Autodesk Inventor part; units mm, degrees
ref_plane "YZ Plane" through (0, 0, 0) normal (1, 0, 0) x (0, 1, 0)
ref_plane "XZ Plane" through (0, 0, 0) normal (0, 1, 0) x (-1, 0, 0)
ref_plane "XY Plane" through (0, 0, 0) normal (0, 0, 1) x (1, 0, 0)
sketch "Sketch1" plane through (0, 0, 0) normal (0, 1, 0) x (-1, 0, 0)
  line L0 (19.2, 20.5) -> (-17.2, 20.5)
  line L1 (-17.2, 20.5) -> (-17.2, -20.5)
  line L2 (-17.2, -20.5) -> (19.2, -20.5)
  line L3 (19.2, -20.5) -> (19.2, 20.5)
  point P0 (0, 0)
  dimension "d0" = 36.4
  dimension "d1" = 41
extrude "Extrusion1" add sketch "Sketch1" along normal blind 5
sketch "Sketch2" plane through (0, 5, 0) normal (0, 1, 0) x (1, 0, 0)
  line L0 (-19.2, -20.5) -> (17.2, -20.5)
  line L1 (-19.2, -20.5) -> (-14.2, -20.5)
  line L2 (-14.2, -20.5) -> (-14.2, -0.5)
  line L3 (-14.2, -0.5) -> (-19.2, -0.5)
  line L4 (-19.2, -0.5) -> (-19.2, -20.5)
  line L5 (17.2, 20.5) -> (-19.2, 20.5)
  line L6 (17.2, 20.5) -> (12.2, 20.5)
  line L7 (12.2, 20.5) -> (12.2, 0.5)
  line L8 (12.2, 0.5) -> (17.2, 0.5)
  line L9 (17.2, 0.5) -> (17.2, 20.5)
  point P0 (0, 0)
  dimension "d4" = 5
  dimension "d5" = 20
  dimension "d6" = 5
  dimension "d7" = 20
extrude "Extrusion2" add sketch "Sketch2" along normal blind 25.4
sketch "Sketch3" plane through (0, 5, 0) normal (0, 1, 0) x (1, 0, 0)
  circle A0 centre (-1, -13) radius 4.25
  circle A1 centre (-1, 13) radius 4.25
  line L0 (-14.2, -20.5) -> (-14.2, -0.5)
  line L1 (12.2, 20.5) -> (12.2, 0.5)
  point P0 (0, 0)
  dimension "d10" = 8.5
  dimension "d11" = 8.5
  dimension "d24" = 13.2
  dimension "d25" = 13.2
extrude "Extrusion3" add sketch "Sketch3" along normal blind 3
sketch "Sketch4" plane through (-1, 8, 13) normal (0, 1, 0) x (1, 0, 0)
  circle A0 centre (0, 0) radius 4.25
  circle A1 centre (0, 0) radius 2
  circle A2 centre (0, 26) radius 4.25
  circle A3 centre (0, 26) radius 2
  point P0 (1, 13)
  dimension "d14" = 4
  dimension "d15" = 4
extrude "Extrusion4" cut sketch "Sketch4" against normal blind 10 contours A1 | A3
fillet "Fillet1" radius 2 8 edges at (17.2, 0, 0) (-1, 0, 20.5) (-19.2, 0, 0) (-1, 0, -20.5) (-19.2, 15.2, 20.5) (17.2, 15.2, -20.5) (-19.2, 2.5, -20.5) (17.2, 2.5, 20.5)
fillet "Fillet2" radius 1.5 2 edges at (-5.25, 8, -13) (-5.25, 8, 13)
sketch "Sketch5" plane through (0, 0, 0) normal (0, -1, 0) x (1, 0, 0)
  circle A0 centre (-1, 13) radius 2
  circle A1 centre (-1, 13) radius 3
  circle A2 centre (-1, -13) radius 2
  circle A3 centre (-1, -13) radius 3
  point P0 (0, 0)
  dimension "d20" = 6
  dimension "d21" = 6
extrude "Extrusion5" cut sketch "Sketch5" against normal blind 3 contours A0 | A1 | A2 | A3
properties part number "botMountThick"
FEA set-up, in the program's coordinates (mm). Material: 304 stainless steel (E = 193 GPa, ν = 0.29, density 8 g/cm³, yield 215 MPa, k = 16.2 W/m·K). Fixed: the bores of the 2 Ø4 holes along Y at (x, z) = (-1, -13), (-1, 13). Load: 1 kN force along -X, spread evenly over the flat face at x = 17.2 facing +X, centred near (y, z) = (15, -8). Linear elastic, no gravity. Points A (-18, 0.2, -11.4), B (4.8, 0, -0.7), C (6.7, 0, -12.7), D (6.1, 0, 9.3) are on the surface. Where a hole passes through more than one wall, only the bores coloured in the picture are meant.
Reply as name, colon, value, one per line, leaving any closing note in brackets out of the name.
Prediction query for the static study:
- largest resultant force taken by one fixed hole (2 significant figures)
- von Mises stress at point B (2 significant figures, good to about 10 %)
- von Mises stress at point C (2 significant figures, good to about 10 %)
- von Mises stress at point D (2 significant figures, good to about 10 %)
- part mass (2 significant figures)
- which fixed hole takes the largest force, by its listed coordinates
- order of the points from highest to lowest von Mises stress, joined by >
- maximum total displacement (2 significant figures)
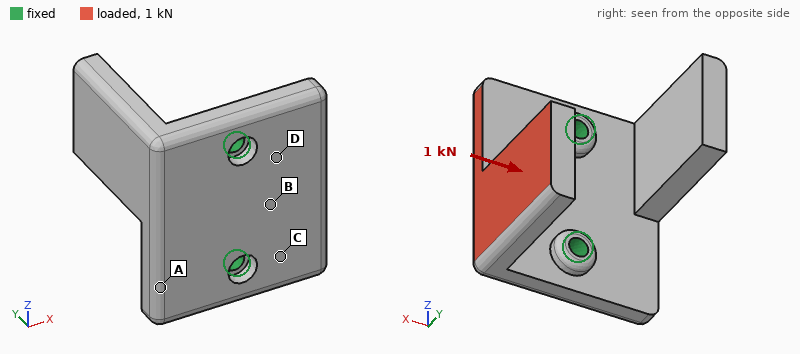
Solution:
largest resultant force taken by one fixed hole: 810 N
von Mises stress at point B: 63 MPa
von Mises stress at point C: 82 MPa
von Mises stress at point D: 43 MPa
part mass: 99 g
which fixed hole takes the largest force, by its listed coordinates: (-1, -13)
order of the points from highest to lowest von Mises stress, joined by >: C > B > D > A
maximum total displacement: 0.16 mm
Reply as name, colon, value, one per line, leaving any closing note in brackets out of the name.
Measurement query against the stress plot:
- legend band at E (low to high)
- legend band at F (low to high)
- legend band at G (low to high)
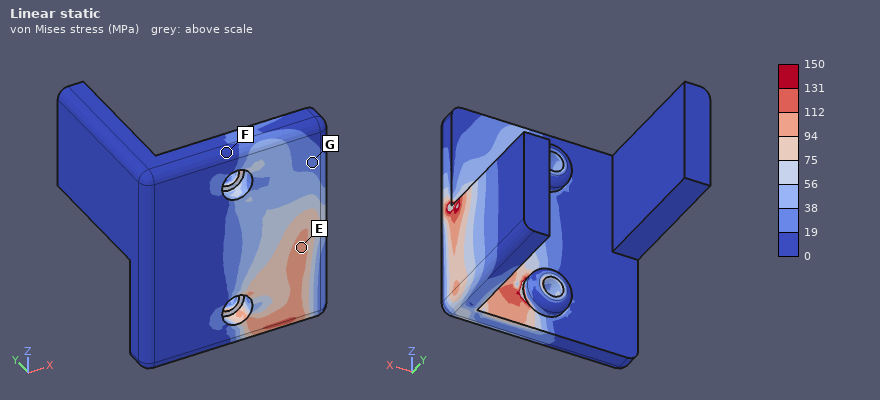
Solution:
legend band at E: 94 to 112 MPa
legend band at F: 0 to 19 MPa
legend band at G: 19 to 38 MPa
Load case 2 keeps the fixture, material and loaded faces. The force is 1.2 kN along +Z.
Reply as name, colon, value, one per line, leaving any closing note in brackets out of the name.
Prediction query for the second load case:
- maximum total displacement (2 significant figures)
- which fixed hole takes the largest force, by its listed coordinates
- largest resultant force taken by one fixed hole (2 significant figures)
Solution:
maximum total displacement: 63 µm
which fixed hole takes the largest force, by its listed coordinates: (-1, -13)
largest resultant force taken by one fixed hole: 1.3 kN
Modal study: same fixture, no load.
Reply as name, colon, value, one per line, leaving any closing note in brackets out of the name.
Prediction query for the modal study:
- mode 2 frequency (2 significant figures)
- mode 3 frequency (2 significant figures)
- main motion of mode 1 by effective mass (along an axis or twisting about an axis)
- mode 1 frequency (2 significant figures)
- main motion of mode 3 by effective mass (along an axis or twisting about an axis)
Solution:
mode 2 frequency: 3100 Hz
mode 3 frequency: 4900 Hz
main motion of mode 1 by effective mass: along X
mode 1 frequency: 2700 Hz
main motion of mode 3 by effective mass: twisting about Y
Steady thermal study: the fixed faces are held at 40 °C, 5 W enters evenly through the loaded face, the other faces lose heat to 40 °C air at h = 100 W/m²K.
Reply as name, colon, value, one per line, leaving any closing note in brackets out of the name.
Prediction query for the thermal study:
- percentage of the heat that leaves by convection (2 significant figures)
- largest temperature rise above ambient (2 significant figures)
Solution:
percentage of the heat that leaves by convection: 70 %
largest temperature rise above ambient: 30 K
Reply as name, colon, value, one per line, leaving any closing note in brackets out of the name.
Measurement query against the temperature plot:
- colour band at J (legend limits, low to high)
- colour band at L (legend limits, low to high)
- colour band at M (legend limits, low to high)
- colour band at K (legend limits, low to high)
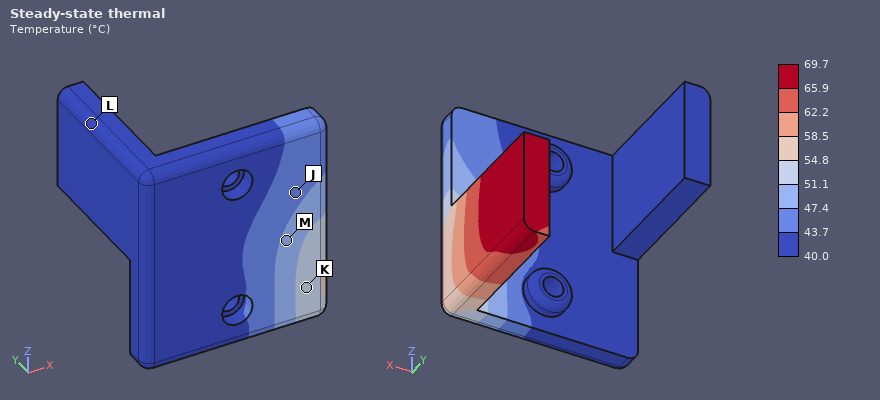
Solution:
colour band at J: 43.7 to 47.4 °C
colour band at L: 40.0 to 43.7 °C
colour band at M: 47.4 to 51.1 °C
colour band at K: 51.1 to 54.8 °C
